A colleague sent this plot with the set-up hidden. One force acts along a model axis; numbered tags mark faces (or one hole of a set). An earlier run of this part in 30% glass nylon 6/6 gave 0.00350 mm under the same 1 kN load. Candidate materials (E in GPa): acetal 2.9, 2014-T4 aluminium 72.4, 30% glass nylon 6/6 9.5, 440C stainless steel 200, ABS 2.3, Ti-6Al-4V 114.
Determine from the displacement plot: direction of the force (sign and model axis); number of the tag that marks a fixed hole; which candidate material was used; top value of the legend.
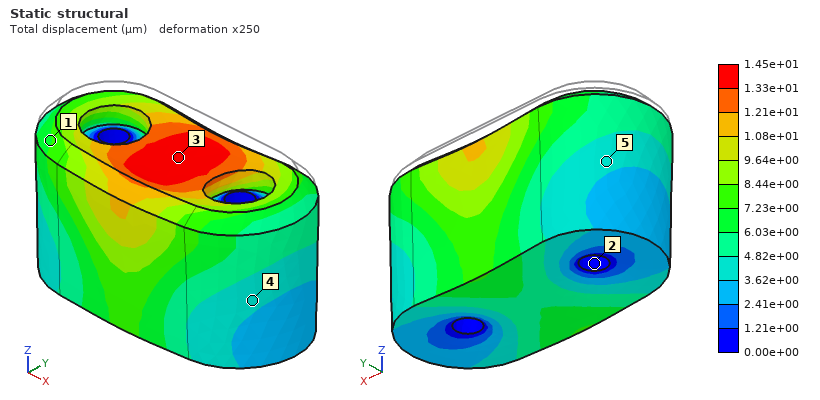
-Z
2
ABS
1.45e+01 µm
